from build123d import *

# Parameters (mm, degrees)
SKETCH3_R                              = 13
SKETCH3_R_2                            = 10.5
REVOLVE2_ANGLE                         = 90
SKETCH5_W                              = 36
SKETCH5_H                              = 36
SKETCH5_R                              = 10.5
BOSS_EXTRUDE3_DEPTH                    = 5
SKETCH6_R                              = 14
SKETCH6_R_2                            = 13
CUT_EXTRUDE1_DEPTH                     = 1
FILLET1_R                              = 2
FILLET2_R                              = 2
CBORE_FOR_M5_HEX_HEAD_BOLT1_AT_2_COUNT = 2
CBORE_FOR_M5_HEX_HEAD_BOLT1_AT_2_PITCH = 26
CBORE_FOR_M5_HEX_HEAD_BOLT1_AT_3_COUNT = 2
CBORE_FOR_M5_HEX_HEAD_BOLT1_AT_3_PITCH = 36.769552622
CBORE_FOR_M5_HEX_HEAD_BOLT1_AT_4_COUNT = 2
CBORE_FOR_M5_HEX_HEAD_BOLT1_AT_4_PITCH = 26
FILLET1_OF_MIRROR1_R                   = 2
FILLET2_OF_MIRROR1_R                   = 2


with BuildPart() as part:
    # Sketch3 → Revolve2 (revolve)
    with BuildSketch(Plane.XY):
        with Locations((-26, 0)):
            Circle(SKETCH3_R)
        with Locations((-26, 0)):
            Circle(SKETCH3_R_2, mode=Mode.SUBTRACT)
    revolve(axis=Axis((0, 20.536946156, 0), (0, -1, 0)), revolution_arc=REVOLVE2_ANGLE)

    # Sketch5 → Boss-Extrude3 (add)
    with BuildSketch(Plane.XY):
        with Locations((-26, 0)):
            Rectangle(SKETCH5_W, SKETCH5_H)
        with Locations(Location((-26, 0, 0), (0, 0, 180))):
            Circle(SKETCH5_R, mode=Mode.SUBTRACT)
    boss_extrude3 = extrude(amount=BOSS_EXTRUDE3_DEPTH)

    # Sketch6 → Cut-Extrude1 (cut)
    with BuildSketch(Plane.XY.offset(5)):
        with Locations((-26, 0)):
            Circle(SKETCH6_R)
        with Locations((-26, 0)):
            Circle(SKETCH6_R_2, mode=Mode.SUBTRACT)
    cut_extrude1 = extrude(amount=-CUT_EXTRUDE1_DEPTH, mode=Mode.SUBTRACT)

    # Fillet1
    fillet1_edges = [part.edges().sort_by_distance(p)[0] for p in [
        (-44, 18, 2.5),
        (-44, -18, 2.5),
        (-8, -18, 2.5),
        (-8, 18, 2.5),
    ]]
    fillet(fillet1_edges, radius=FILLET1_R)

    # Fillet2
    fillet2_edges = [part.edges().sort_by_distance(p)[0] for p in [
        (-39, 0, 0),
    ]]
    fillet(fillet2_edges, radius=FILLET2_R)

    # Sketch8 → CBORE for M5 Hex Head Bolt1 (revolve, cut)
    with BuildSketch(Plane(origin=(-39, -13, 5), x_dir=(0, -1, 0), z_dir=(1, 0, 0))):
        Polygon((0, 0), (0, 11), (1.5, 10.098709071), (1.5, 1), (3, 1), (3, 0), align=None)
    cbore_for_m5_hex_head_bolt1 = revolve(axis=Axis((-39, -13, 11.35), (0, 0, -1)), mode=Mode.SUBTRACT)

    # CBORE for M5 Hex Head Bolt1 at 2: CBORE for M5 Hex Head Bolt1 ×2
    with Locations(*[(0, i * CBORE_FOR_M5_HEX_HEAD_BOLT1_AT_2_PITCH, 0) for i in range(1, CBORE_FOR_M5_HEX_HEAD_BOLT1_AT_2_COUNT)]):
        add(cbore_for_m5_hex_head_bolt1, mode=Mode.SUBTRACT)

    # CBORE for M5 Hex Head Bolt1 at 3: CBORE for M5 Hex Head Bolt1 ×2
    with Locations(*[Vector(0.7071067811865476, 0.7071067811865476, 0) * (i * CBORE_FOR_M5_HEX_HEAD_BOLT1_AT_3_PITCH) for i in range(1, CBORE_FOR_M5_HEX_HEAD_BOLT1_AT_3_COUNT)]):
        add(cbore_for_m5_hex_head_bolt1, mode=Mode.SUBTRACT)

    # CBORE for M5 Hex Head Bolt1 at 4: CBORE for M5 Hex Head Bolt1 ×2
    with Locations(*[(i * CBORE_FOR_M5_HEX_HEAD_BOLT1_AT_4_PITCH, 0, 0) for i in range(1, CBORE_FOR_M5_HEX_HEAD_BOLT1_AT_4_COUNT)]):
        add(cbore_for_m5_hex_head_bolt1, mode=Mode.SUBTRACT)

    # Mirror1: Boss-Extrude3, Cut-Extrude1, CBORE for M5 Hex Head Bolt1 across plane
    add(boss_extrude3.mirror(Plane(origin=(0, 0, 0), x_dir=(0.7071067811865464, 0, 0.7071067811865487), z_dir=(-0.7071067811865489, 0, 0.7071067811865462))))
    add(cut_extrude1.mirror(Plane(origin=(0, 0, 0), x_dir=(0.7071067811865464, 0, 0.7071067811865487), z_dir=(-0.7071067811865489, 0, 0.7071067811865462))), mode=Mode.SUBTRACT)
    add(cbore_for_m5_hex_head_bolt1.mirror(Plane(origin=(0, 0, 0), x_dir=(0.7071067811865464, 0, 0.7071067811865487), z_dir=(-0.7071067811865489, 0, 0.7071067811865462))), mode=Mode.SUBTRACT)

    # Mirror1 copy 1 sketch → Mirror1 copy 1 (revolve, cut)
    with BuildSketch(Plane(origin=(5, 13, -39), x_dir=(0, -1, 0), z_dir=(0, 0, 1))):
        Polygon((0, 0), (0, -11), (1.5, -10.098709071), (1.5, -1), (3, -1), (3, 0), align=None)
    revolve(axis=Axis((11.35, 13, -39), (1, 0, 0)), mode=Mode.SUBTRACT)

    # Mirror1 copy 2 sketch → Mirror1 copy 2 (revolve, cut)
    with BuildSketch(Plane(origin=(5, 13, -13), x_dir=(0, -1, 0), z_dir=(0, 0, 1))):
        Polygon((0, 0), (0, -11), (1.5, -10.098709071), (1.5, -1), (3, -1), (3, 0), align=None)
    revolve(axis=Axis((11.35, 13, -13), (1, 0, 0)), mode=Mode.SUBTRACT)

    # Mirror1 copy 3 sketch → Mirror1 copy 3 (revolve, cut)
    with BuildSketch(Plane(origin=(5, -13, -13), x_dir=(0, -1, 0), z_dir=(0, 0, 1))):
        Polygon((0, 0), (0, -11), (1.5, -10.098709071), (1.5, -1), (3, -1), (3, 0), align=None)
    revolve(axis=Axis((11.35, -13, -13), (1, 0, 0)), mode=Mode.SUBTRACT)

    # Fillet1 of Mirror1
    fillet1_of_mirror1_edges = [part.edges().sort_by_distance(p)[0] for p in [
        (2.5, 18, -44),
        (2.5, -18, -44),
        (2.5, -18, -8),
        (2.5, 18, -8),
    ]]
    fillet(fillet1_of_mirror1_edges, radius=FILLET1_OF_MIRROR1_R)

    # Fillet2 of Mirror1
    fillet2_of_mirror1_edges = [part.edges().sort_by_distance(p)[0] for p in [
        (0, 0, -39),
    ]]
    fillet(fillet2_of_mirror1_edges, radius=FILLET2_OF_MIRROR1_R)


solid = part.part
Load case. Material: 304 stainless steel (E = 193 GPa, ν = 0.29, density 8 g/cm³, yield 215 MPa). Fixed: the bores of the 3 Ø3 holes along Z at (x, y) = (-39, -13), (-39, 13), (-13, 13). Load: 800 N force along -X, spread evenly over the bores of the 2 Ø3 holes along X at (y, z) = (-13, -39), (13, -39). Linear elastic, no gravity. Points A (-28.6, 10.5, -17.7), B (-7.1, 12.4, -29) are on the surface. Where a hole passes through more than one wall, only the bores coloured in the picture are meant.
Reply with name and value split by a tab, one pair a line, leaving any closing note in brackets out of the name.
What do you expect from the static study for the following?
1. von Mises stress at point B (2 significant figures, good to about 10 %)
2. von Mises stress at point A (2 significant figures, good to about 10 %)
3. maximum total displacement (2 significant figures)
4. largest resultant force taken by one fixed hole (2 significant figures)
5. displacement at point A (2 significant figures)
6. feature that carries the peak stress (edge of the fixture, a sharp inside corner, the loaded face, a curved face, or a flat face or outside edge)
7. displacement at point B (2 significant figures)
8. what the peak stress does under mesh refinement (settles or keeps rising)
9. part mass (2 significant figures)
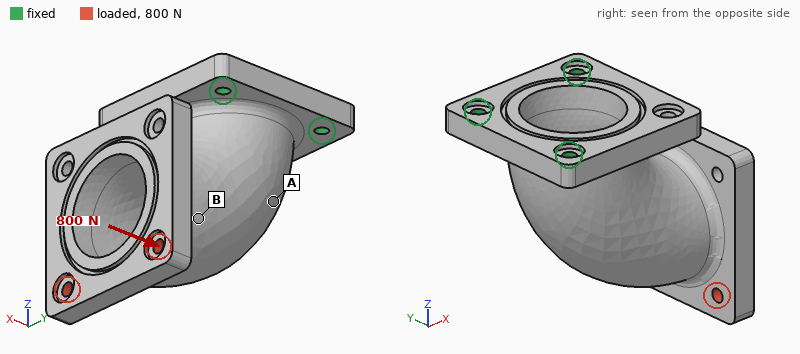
von Mises stress at point B	16 MPa
von Mises stress at point A	32 MPa
maximum total displacement	77 µm
largest resultant force taken by one fixed hole	1.3 kN
displacement at point A	17 µm
feature that carries the peak stress	edge of the fixture
displacement at point B	39 µm
what the peak stress does under mesh refinement	keeps rising
part mass	130 g
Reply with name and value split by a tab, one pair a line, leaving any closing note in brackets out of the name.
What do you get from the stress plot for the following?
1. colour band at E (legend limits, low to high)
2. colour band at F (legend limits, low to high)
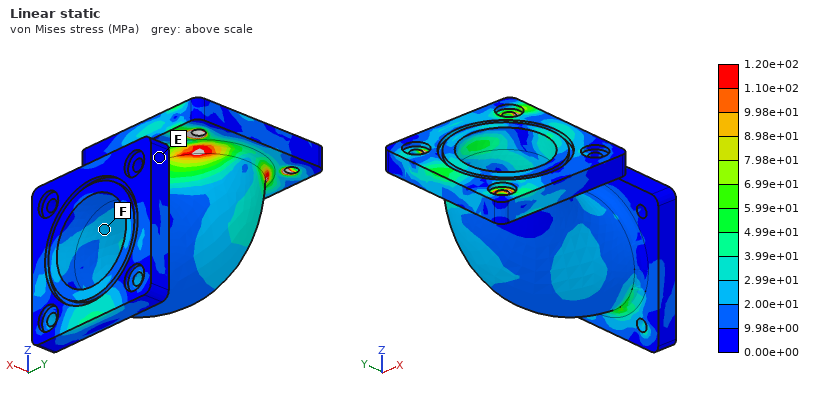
colour band at E	0.00e+00 to 9.98e+00 MPa
colour band at F	2.00e+01 to 2.99e+01 MPa
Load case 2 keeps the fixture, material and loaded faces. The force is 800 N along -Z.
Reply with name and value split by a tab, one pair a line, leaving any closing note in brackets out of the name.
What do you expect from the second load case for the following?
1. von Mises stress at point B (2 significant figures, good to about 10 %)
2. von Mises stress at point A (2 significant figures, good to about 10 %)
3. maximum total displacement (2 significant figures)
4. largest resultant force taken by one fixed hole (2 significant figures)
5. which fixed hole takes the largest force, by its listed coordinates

von Mises stress at point B	14 MPa
von Mises stress at point A	24 MPa
maximum total displacement	61 µm
largest resultant force taken by one fixed hole	1.2 kN
which fixed hole takes the largest force, by its listed coordinates	(-13, 13)
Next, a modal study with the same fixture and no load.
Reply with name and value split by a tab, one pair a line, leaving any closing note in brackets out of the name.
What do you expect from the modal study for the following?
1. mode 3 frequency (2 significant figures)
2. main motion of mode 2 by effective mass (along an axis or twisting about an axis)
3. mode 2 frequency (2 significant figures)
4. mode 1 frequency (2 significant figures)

mode 3 frequency	8300 Hz
main motion of mode 2 by effective mass	along Y
mode 2 frequency	3600 Hz
mode 1 frequency	2400 Hz
